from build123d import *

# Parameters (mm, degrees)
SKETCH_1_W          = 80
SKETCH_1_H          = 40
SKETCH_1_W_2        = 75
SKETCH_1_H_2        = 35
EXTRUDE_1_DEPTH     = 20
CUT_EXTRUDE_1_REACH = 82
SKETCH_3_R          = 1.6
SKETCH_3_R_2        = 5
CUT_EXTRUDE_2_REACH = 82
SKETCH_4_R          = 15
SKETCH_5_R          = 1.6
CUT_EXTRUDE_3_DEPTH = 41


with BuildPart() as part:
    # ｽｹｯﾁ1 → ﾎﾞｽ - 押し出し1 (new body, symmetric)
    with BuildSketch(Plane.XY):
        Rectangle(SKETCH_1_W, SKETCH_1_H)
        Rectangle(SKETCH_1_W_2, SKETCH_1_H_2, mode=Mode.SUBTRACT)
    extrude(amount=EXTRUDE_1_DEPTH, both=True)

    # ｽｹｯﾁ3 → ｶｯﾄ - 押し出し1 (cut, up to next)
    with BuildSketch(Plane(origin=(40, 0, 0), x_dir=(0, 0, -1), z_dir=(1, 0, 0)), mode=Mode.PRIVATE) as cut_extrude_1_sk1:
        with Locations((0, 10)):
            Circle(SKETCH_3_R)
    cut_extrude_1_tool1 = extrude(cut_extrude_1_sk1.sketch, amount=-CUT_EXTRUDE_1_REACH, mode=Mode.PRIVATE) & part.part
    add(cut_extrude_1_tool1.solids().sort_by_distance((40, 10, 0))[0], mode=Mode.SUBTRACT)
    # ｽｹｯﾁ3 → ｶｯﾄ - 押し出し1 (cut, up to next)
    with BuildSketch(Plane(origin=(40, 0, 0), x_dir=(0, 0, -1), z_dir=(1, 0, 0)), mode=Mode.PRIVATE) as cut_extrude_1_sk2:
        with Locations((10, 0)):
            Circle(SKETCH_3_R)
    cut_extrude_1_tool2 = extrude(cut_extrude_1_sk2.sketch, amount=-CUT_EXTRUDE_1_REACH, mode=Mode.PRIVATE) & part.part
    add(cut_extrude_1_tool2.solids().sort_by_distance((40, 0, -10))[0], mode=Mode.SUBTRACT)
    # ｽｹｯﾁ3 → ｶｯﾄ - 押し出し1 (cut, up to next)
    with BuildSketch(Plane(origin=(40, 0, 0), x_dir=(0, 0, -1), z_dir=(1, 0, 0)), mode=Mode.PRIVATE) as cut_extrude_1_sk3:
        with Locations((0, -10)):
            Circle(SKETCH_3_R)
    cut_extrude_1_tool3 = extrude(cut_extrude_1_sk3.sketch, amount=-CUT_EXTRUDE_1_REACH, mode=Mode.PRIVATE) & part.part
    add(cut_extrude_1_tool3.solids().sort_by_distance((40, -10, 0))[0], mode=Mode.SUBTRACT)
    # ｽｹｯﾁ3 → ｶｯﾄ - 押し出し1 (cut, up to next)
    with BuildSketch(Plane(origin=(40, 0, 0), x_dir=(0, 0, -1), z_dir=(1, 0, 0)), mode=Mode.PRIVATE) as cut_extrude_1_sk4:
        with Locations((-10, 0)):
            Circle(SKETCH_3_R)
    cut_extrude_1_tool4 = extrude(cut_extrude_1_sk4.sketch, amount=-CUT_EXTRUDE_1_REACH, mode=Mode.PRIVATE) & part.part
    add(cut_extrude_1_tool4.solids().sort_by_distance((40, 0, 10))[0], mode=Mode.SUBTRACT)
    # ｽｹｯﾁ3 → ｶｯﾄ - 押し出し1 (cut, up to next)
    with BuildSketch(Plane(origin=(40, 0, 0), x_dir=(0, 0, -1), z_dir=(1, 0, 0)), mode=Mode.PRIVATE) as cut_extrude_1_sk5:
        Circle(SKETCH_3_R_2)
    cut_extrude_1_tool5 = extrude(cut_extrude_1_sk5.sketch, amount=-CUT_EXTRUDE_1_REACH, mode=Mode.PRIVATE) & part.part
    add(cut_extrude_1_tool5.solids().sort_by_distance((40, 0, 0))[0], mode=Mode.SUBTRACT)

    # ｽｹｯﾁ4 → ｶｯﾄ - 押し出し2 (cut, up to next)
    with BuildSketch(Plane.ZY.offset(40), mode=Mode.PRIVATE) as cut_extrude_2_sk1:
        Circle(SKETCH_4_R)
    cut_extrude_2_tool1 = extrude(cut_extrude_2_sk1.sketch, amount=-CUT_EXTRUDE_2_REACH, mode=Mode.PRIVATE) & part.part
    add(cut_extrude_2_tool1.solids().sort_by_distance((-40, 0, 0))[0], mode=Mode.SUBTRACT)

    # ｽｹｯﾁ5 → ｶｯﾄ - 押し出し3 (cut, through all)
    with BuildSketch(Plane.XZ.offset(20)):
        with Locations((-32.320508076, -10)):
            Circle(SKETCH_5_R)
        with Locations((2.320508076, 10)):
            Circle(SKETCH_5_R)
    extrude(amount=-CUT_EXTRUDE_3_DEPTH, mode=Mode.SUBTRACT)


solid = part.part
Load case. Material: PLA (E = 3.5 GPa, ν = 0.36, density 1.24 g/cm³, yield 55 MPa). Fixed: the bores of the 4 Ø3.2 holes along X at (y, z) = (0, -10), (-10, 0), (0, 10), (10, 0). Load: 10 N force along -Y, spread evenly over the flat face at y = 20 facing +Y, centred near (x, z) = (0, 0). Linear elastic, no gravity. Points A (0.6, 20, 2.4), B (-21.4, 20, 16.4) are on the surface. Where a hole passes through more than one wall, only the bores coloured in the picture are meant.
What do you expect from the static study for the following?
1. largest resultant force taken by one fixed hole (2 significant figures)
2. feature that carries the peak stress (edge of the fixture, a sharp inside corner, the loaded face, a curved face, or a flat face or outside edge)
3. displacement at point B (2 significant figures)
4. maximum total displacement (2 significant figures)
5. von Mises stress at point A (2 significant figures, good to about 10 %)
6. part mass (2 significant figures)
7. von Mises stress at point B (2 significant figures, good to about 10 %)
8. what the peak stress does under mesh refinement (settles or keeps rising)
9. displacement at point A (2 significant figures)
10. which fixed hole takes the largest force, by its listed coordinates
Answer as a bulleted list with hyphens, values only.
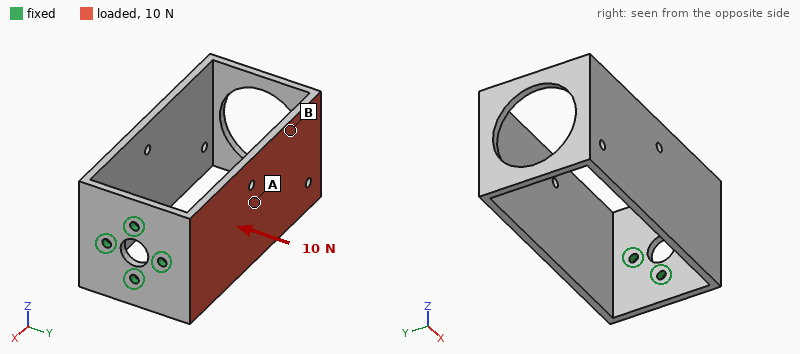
- 14 N
- edge of the fixture
- 0.89 mm
- 1.0 mm
- 0.84 MPa
- 26 g
- 1.7 MPa
- keeps rising
- 0.59 mm
- (10, 0)
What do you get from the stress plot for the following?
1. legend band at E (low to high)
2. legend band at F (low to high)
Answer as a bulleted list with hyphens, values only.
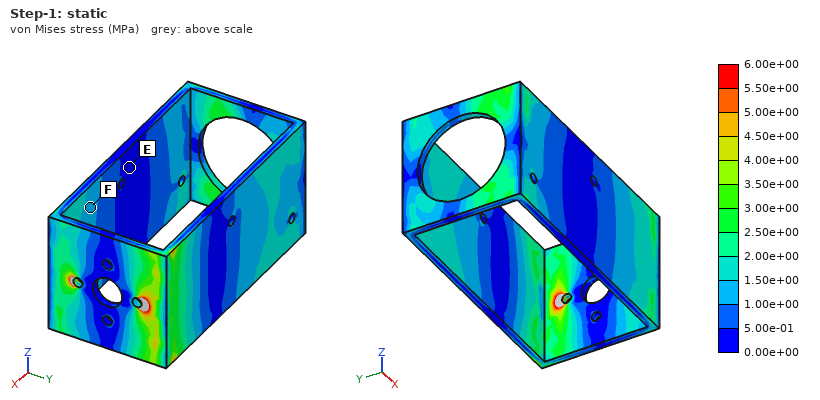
- 0.00e+00 to 5.00e-01 MPa
- 1.00e+00 to 1.50e+00 MPa
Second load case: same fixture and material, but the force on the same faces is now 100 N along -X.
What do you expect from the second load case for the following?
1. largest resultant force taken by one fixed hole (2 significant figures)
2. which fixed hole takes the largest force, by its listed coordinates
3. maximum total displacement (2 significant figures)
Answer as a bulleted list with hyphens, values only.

- 120 N
- (10, 0)
- 1.1 mm
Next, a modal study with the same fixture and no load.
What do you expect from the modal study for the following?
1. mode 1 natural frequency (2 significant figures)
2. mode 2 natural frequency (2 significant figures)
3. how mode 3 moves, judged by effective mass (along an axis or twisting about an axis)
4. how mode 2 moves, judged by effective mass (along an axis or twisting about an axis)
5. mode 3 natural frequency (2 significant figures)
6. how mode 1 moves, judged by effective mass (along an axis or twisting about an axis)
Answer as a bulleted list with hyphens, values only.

- 120 Hz
- 200 Hz
- twisting about X
- along Z
- 320 Hz
- along Y
